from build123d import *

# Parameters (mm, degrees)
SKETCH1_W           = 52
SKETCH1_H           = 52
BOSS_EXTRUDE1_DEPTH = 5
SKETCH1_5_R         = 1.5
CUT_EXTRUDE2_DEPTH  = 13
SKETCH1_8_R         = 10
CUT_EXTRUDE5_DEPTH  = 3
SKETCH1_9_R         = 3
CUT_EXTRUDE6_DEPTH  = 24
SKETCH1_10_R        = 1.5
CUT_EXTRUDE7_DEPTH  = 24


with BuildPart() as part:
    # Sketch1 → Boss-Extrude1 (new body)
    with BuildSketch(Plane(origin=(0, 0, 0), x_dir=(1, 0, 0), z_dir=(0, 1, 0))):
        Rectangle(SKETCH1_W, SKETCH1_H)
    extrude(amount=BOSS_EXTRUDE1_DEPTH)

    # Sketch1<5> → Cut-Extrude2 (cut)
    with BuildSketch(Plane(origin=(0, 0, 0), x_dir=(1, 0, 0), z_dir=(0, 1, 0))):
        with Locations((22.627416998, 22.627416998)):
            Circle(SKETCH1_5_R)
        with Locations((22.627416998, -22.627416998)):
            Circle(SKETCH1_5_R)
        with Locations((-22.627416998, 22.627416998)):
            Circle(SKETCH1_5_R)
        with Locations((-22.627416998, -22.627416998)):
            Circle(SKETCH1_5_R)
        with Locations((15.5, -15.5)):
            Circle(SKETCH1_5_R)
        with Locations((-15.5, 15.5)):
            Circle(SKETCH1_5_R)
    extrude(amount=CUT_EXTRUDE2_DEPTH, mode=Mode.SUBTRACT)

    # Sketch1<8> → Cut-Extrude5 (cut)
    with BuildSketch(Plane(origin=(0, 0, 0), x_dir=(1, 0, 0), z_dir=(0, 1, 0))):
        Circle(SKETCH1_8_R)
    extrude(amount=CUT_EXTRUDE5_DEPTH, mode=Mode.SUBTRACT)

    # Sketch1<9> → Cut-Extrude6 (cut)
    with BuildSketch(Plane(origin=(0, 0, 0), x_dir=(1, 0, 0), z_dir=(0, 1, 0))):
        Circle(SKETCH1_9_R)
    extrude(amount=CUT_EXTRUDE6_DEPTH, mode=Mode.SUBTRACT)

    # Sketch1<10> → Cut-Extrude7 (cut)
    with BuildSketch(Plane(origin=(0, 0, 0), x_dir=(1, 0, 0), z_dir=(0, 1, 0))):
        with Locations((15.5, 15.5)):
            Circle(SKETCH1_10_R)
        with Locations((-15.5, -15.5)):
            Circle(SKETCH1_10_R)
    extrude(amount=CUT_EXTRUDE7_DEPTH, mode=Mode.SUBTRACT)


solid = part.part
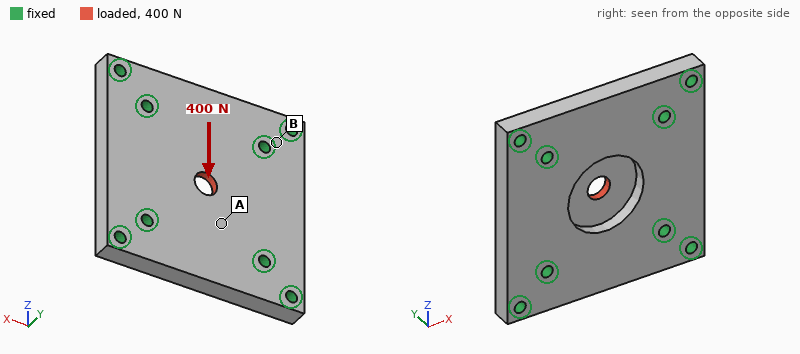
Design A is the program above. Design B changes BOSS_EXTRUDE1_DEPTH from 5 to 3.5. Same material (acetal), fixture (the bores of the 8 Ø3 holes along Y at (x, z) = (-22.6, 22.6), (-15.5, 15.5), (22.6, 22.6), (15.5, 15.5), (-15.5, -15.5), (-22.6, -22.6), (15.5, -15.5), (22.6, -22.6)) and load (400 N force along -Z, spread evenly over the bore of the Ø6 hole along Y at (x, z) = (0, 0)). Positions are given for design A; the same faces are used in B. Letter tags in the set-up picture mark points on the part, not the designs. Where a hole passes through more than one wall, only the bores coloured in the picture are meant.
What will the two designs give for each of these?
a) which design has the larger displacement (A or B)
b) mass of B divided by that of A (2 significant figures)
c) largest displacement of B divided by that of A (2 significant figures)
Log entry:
B
0.68
3.4
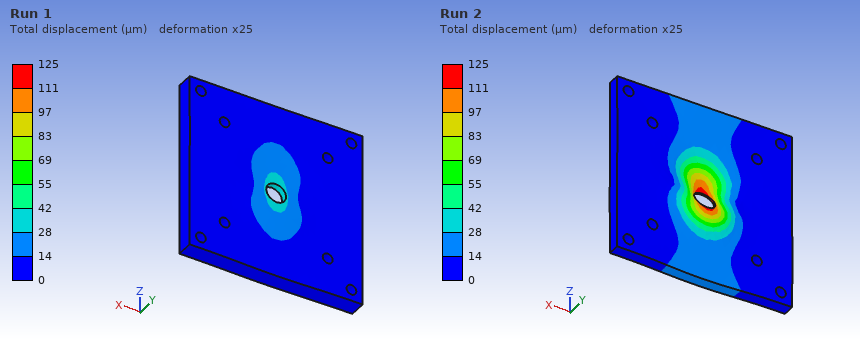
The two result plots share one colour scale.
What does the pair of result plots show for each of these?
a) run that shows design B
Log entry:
Run 2
